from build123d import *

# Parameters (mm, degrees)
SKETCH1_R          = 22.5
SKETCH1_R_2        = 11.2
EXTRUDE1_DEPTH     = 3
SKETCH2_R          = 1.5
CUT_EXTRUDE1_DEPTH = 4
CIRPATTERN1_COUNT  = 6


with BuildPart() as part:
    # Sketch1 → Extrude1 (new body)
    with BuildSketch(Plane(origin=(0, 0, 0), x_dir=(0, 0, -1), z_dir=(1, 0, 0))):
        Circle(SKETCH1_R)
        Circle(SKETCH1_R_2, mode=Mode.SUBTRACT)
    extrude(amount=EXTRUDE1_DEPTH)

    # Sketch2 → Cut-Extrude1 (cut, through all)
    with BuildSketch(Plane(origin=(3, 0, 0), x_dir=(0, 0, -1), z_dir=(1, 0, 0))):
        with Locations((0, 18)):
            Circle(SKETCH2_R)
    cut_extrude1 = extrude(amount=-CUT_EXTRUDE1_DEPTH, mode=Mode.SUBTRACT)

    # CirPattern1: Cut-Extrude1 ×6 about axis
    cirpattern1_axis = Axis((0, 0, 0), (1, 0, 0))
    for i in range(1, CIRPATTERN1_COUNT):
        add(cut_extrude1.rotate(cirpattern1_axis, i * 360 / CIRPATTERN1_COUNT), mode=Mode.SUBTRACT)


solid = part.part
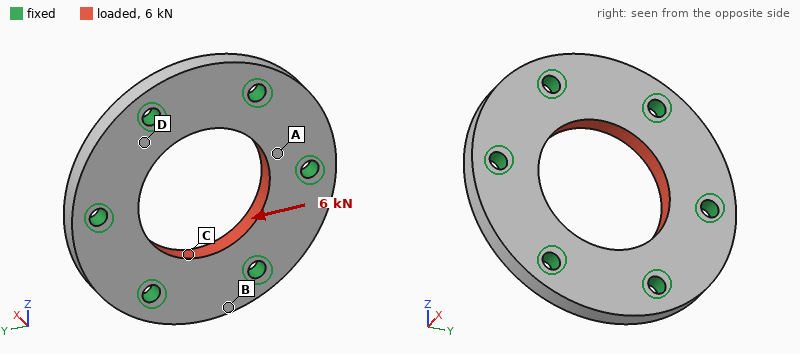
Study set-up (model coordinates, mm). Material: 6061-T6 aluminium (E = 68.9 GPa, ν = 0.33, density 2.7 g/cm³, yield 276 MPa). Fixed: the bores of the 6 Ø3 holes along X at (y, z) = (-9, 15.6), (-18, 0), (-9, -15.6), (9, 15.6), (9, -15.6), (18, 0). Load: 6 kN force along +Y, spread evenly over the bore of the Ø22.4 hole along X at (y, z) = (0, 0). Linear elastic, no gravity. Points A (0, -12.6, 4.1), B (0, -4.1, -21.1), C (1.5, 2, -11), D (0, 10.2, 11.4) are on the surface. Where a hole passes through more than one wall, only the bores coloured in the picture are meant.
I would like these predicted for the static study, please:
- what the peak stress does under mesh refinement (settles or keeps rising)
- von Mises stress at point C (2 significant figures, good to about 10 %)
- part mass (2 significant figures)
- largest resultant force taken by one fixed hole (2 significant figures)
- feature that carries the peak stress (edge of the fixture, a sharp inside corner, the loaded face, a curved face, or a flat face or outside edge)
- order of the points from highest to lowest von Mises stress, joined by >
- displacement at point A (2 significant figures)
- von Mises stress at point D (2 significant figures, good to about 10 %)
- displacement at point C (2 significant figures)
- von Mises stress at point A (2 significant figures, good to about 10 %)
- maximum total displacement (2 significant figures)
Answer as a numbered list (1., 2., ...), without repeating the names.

1. keeps rising
2. 49 MPa
3. 9.3 g
4. 1.3 kN
5. edge of the fixture
6. C > A > D > B
7. 4.4 µm
8. 19 MPa
9. 4.7 µm
10. 36 MPa
11. 6.2 µm
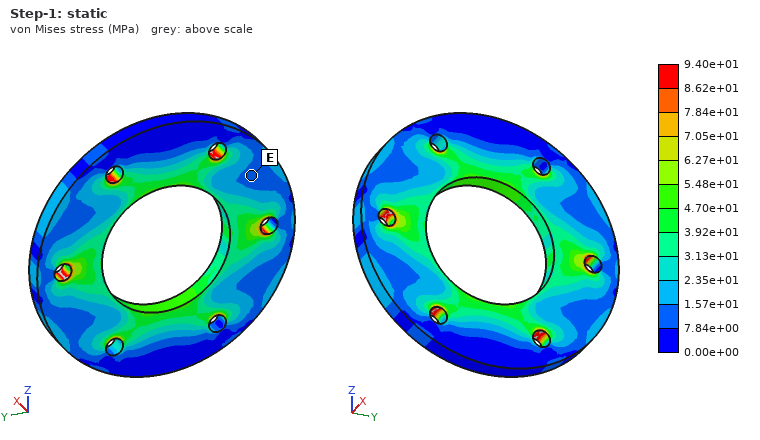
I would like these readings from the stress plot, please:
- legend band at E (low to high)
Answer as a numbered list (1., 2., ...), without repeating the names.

1. 7.84e+00 to 1.57e+01 MPa
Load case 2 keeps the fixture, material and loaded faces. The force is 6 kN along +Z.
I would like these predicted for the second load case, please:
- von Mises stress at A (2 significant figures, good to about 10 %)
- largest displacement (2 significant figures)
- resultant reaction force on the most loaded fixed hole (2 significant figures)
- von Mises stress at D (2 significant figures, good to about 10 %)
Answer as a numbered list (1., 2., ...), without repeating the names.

1. 29 MPa
2. 6.3 µm
3. 1.2 kN
4. 39 MPa
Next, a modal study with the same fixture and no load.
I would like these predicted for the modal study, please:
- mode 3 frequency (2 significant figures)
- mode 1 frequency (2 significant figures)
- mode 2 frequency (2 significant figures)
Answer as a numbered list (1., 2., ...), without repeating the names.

1. 37 kHz
2. 36 kHz
3. 37 kHz
